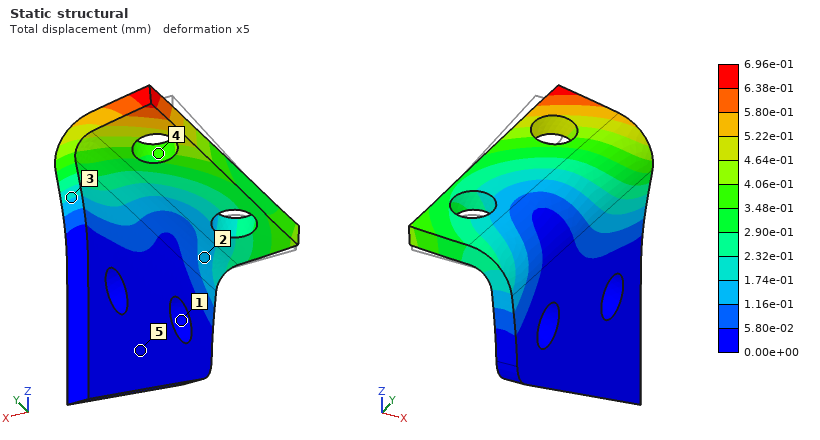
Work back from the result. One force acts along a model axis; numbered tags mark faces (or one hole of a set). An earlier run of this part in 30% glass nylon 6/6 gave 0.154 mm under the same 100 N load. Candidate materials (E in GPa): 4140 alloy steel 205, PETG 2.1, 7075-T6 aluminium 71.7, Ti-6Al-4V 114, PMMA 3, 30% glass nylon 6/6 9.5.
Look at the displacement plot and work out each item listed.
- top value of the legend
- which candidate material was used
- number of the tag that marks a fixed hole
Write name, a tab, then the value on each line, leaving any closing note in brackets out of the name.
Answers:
top value of the legend	6.96e-01 mm
which candidate material was used	PETG
number of the tag that marks a fixed hole	1
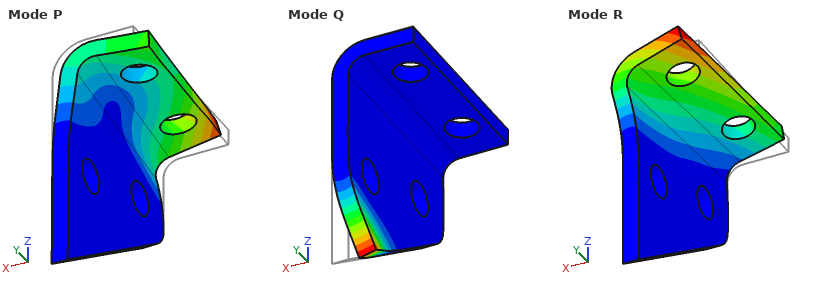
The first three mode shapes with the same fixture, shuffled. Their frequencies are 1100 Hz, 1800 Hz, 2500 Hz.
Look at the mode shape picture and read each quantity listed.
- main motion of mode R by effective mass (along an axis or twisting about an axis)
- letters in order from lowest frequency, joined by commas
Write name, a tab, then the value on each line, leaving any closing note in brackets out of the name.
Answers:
main motion of mode R by effective mass	along X
letters in order from lowest frequency, joined by commas	R, P, Q
